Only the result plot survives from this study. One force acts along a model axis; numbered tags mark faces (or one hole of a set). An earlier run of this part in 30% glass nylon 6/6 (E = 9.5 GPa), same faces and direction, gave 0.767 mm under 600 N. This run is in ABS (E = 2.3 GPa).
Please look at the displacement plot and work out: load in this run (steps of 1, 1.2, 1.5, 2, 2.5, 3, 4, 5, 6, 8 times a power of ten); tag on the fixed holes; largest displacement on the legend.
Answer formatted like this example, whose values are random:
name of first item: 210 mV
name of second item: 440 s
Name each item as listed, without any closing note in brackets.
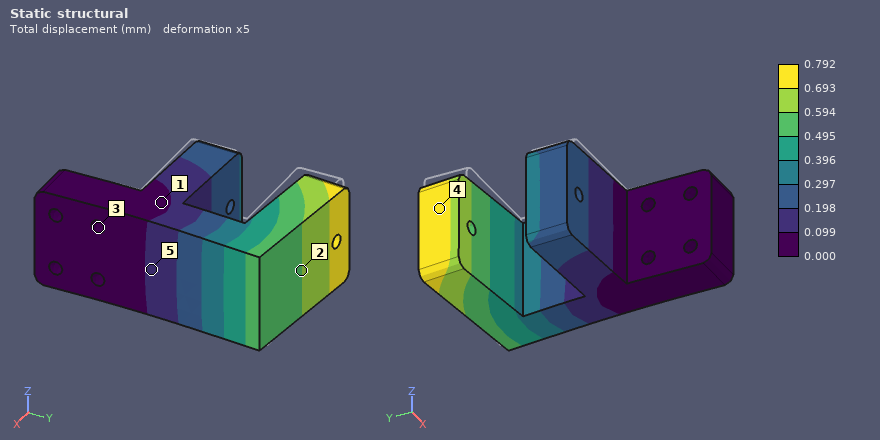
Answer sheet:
load in this run: 150 N
tag on the fixed holes: 3
largest displacement on the legend: 0.792 mm
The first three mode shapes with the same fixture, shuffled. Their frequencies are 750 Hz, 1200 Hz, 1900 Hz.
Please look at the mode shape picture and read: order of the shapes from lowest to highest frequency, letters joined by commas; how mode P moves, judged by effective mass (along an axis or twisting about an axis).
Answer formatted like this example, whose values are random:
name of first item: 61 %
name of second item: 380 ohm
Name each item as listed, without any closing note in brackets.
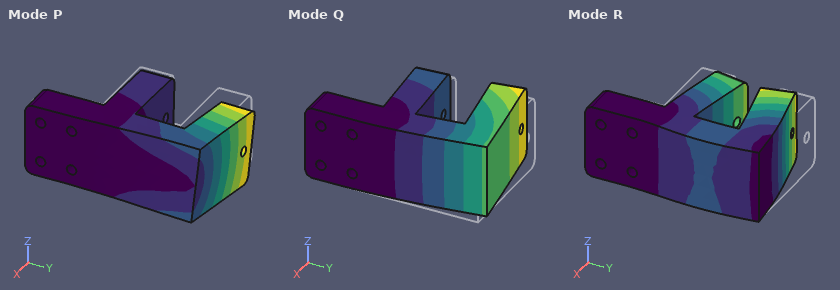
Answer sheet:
order of the shapes from lowest to highest frequency, letters joined by commas: Q, P, R
how mode P moves, judged by effective mass: along Z
